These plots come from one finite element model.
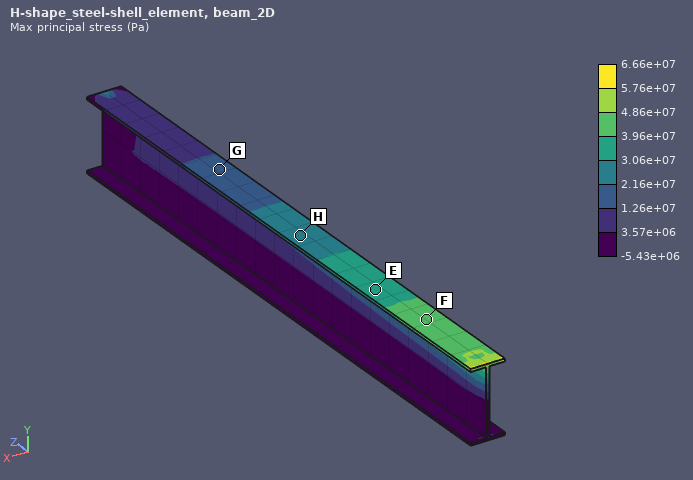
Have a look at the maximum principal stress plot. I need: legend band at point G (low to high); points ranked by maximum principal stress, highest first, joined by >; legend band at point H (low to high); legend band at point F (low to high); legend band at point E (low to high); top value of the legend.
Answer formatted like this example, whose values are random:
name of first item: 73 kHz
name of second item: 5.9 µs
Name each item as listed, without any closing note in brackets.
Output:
legend band at point G: 1.26e+07 to 2.16e+07 Pa
points ranked by maximum principal stress, highest first, joined by >: F > E > H > G
legend band at point H: 2.16e+07 to 3.06e+07 Pa
legend band at point F: 3.96e+07 to 4.86e+07 Pa
legend band at point E: 3.06e+07 to 3.96e+07 Pa
top value of the legend: 6.66e+07 Pa
